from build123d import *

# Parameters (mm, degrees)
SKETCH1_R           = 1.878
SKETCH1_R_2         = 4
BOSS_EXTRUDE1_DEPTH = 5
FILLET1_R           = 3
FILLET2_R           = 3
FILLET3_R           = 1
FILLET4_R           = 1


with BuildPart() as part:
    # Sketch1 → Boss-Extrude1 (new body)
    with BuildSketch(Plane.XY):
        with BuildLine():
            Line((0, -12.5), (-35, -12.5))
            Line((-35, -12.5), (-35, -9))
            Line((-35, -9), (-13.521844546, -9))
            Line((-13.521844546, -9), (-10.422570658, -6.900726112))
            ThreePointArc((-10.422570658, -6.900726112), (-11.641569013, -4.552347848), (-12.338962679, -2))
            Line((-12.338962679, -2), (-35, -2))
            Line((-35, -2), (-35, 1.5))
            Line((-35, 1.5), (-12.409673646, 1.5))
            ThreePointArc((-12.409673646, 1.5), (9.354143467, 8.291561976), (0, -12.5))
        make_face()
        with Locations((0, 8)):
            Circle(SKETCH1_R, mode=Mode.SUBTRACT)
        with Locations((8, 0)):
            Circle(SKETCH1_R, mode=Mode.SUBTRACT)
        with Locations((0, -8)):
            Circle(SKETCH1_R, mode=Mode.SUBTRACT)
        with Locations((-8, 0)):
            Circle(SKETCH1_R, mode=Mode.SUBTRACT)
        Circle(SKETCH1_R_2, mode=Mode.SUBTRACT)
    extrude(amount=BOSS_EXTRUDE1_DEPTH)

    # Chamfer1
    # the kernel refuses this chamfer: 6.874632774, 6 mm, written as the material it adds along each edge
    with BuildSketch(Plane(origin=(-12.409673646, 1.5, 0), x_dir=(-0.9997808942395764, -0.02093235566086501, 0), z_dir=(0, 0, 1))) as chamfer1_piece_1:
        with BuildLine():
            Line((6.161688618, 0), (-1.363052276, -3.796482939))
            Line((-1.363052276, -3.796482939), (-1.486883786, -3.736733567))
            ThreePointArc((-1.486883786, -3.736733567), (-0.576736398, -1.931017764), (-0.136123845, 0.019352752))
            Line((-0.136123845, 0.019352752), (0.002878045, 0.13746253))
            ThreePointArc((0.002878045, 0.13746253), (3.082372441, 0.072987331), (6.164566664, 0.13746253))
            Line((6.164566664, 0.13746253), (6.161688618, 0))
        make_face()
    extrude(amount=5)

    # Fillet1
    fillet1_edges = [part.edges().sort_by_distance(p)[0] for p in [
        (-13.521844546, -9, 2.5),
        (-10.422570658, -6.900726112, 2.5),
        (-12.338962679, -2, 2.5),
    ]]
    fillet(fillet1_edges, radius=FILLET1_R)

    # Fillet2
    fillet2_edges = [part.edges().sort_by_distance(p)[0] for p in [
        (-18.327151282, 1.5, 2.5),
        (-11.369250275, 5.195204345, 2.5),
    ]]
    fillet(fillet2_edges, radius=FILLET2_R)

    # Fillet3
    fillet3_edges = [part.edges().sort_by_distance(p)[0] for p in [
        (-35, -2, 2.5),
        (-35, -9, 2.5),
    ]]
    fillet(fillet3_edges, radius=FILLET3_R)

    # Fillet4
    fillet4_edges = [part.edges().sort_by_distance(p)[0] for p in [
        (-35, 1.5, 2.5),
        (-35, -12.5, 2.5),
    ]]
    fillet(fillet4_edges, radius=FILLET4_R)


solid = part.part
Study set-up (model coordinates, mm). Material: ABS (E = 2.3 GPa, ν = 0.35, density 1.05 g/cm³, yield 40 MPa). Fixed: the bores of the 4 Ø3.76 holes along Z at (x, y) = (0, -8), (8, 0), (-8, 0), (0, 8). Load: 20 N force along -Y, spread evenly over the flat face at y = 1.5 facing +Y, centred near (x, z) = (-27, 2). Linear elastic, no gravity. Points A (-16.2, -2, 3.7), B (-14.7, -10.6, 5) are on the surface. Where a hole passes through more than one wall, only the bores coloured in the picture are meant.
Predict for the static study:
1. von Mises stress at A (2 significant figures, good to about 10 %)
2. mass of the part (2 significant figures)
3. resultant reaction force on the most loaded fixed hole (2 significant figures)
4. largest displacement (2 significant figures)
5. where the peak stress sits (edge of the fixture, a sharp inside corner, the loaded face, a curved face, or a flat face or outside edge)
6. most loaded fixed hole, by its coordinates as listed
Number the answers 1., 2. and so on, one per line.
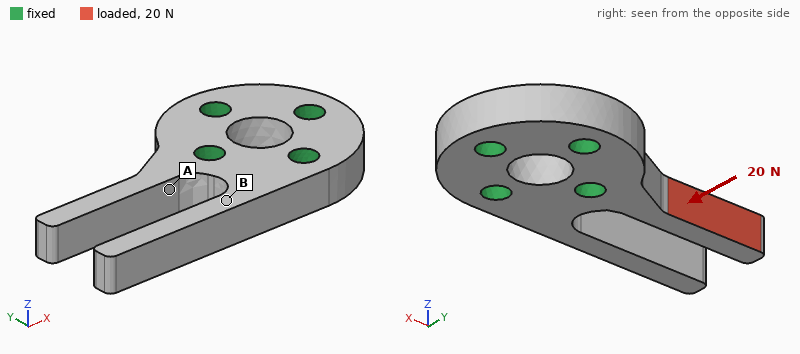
1. 13 MPa
2. 3.1 g
3. 23 N
4. 0.58 mm
5. a curved face
6. (0, 8)
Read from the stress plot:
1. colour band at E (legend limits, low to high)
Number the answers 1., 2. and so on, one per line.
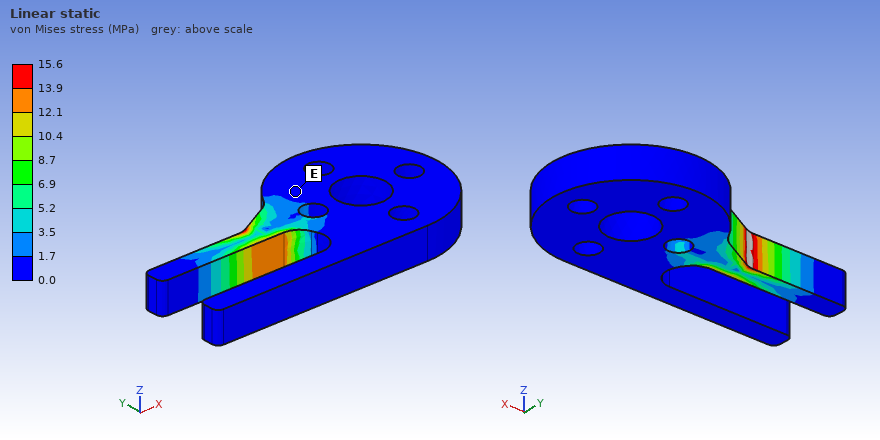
1. 0.0 to 1.7 MPa
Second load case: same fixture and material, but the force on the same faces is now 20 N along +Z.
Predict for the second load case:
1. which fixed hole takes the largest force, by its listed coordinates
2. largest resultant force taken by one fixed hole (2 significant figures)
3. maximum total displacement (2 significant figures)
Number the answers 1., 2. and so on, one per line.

1. (-8, 0)
2. 30 N
3. 0.52 mm
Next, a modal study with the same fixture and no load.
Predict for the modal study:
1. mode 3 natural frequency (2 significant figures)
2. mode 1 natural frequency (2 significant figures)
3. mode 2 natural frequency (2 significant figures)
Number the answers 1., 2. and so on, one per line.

1. 2100 Hz
2. 1400 Hz
3. 1500 Hz
